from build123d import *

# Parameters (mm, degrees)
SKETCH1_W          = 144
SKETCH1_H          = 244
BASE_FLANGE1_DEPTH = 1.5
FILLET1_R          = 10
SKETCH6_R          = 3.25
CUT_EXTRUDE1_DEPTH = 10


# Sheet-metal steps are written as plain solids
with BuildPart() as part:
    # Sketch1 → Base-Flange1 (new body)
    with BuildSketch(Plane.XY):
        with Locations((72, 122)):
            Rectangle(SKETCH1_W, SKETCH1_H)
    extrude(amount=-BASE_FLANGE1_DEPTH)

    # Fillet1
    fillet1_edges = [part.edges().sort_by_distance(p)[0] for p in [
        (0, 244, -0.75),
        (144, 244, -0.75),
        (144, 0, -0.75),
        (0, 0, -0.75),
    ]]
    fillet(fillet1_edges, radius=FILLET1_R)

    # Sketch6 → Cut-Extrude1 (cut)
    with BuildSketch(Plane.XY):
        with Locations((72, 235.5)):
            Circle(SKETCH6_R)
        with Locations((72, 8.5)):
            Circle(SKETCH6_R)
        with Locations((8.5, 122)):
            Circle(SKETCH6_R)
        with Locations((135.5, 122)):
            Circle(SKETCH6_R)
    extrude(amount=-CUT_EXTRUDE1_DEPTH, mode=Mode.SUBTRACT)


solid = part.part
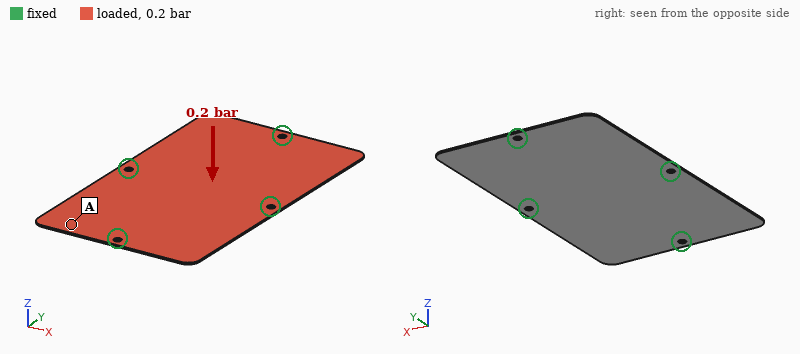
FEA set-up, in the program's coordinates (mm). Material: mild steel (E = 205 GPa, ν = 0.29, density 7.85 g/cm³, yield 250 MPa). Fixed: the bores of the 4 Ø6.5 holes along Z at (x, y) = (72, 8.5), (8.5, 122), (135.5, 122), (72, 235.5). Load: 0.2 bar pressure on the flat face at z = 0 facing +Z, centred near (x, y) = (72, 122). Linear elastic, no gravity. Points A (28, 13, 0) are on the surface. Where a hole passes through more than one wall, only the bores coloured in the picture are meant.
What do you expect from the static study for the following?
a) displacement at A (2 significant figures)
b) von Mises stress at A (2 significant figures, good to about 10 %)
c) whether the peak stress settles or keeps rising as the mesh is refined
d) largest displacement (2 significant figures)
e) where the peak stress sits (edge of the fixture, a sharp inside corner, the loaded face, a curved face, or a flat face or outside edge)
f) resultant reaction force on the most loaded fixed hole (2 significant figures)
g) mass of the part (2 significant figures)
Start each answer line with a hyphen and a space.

- 0.36 mm
- 19 MPa
- keeps rising
- 0.65 mm
- edge of the fixture
- 180 N
- 410 g
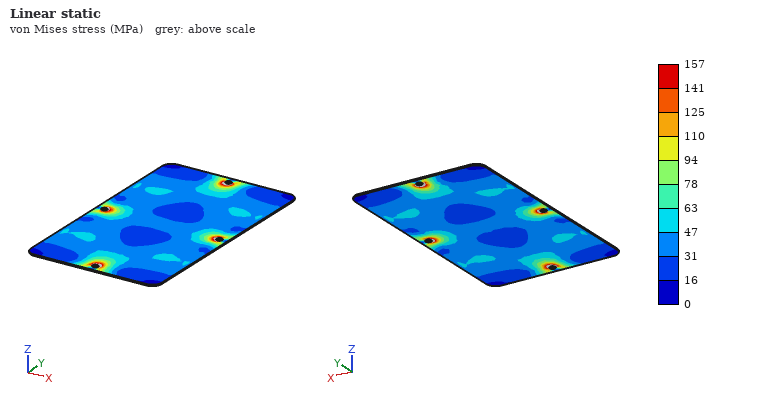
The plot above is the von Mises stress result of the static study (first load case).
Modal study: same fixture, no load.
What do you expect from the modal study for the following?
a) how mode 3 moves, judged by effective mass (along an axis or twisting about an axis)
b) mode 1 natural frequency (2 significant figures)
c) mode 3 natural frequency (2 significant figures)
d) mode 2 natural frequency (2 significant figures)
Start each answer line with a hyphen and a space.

- twisting about X
- 290 Hz
- 320 Hz
- 290 Hz
